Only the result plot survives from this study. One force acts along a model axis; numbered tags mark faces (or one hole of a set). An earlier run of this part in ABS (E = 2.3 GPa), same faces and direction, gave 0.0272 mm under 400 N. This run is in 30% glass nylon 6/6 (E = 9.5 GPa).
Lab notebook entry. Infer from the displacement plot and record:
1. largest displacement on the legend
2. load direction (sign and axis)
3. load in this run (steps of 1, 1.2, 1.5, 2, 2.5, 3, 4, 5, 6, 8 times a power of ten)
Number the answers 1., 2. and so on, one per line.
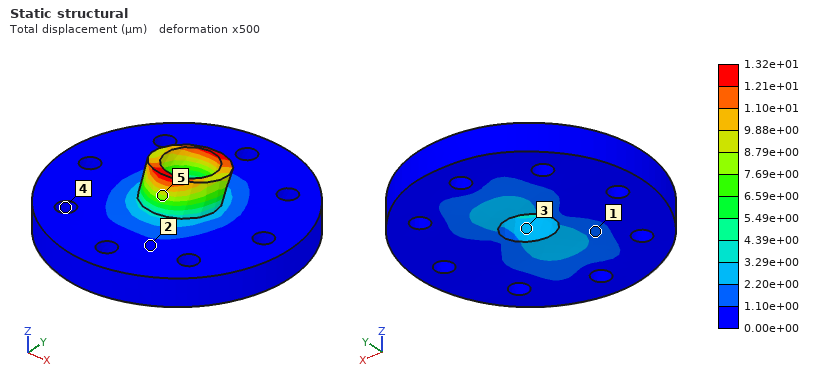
1. 1.32e+01 µm
2. +Y
3. 800 N
